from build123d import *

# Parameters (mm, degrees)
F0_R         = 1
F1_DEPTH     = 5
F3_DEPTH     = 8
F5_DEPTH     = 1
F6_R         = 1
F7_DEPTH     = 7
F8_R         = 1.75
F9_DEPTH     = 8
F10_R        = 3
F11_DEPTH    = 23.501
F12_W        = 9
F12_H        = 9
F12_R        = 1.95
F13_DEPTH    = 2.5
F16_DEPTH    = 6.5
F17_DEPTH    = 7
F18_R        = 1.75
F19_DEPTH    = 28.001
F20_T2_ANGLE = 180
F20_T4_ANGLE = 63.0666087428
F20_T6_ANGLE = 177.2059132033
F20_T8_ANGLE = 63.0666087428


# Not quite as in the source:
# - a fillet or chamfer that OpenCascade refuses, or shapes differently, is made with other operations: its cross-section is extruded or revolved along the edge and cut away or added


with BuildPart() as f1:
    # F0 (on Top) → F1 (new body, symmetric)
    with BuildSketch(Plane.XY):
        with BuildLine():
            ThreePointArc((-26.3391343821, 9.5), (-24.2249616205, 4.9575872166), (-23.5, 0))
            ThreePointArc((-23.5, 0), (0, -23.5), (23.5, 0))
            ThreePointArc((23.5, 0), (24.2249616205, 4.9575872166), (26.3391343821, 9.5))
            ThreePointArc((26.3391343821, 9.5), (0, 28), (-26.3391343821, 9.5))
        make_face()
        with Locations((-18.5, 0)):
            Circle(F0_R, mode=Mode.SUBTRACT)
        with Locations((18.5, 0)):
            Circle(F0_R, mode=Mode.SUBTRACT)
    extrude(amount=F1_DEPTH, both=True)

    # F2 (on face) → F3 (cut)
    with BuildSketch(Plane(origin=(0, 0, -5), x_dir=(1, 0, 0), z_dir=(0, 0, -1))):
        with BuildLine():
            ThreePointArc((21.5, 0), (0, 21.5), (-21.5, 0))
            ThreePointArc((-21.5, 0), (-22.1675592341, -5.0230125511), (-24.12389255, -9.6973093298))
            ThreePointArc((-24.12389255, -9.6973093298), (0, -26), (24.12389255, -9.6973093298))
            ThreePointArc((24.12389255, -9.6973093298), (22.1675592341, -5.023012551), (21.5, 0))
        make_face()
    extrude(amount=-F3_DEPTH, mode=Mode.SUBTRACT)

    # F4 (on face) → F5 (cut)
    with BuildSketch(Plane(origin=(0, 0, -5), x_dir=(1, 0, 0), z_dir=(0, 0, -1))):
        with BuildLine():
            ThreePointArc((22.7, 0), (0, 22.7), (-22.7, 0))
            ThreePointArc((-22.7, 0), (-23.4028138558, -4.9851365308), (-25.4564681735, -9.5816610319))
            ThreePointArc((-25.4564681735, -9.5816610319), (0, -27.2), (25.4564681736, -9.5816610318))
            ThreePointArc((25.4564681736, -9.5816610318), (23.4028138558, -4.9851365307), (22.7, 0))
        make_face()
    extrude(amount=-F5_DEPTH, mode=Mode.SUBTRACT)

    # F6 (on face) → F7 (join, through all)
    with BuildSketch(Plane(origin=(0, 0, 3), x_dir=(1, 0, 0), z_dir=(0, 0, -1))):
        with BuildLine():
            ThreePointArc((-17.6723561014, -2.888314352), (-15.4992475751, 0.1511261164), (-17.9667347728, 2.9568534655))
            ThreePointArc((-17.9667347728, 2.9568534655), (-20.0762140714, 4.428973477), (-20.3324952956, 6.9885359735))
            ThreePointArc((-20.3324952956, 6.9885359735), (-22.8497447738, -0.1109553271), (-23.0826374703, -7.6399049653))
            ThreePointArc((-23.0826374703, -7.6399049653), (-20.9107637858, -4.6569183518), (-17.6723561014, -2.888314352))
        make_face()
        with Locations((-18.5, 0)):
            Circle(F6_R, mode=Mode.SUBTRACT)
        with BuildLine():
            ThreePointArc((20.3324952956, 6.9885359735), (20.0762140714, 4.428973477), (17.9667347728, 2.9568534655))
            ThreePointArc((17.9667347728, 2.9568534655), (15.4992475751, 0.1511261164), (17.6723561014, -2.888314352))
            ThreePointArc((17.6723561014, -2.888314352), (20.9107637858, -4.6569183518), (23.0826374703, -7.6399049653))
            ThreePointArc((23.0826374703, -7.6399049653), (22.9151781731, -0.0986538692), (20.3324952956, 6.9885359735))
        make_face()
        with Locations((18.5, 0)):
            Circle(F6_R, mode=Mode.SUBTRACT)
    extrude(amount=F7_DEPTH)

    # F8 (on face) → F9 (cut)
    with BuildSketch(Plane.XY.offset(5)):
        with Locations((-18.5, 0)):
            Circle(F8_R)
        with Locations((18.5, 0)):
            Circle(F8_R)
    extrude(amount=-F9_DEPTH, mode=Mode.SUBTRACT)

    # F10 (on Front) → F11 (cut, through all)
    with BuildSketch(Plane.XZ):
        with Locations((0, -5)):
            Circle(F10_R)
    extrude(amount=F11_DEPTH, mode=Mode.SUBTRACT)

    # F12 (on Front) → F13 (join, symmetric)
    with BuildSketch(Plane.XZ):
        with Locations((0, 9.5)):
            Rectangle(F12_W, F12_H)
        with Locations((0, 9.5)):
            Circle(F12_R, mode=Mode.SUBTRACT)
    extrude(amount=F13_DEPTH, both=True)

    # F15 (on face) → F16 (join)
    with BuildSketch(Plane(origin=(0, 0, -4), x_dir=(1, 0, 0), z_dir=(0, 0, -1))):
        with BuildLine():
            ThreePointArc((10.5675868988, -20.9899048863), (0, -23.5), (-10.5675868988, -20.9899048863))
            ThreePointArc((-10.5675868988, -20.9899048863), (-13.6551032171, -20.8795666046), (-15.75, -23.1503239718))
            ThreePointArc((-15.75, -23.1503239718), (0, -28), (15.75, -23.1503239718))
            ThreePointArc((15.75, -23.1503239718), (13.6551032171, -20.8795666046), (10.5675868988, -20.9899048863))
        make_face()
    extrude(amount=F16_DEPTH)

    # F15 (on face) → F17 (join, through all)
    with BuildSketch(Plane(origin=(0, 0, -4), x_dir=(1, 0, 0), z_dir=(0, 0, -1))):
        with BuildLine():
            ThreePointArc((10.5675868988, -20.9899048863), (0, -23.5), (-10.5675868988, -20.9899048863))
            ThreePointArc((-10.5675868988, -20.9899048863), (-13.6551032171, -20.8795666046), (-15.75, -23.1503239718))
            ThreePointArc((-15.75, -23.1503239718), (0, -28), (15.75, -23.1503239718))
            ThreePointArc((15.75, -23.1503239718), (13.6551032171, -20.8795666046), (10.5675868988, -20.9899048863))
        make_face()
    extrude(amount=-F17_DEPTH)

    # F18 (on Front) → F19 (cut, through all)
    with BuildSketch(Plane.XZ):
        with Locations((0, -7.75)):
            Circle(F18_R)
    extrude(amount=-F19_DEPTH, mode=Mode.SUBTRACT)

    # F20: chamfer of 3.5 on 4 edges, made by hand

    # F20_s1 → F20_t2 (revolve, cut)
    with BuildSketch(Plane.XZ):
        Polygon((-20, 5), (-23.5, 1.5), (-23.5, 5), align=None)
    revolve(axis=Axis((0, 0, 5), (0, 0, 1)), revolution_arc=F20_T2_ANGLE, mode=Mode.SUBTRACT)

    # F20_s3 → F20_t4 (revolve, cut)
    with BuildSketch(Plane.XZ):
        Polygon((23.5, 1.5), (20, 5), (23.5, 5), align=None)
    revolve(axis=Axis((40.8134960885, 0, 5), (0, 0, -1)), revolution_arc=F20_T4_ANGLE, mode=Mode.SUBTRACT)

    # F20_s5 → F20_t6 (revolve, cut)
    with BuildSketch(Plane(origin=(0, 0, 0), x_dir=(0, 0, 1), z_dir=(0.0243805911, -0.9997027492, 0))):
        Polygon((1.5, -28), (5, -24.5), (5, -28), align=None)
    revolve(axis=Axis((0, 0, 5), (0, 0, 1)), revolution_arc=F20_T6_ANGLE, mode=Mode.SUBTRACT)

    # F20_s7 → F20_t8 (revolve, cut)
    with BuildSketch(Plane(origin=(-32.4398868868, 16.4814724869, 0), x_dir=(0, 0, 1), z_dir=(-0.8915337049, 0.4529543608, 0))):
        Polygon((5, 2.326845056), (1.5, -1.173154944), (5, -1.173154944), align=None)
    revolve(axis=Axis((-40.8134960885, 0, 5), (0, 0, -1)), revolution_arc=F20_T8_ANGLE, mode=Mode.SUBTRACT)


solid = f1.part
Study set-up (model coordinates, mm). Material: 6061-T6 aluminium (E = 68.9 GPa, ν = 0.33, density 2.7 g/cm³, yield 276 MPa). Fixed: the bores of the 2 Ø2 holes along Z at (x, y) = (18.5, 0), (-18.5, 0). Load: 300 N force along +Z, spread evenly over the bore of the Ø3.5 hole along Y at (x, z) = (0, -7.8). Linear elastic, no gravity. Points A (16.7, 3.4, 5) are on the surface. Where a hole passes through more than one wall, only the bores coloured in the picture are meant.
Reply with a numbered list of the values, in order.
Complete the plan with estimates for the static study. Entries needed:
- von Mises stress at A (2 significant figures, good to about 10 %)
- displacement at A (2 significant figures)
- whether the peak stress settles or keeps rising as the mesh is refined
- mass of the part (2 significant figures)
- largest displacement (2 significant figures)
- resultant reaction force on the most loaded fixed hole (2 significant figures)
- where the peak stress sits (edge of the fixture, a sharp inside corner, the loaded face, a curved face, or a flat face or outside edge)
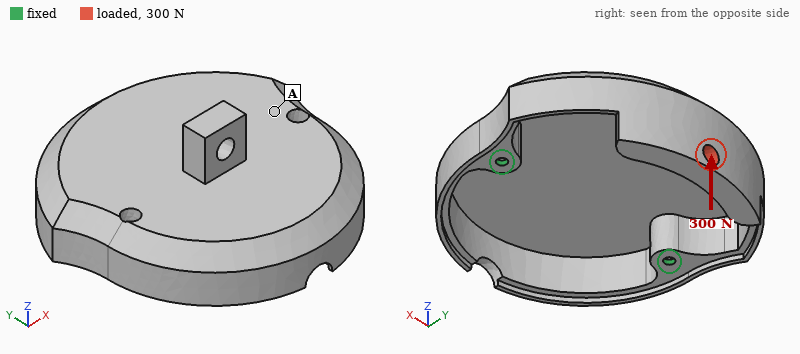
1. 64 MPa
2. 0.22 mm
3. keeps rising
4. 20 g
5. 0.93 mm
6. 150 N
7. edge of the fixture
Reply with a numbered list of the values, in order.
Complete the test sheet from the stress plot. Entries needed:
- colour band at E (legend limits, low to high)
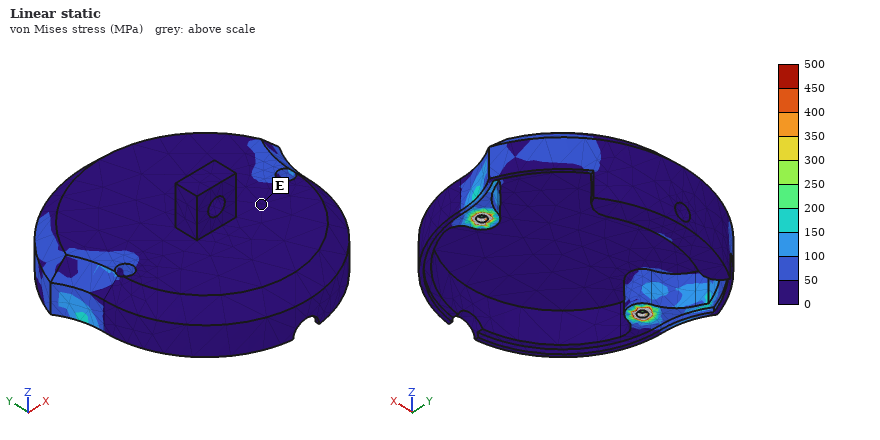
1. 0 to 50 MPa
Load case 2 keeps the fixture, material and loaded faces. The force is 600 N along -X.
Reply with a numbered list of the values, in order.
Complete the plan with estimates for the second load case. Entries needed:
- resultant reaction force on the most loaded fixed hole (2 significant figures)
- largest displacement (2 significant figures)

1. 460 N
2. 0.22 mm
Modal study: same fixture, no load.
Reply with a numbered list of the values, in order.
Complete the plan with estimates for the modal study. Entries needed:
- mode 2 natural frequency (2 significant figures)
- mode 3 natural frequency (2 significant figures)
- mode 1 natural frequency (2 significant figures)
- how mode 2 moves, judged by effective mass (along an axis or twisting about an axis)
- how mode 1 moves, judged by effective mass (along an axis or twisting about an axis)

1. 3400 Hz
2. 3800 Hz
3. 1100 Hz
4. along X
5. along Z
